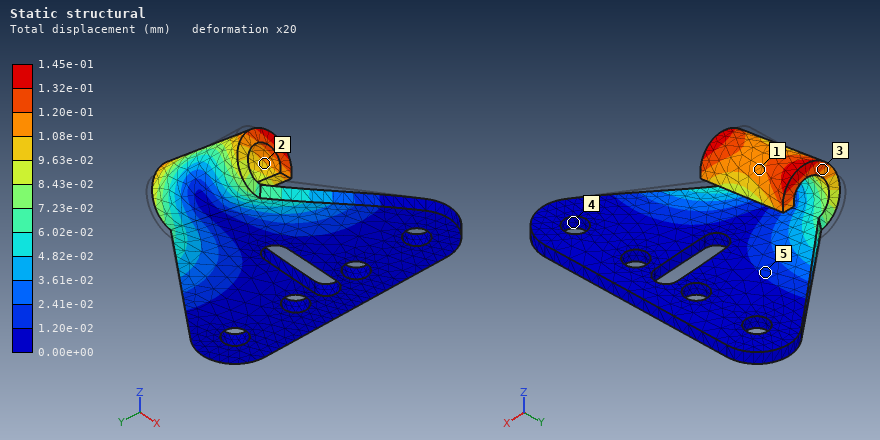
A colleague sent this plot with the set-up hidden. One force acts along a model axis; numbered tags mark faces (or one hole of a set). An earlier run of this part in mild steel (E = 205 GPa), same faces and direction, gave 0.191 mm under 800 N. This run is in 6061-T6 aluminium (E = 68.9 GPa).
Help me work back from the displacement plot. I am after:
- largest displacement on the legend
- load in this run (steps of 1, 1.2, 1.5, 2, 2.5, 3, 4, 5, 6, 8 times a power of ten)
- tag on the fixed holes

1.45e-01 mm
200 N
4
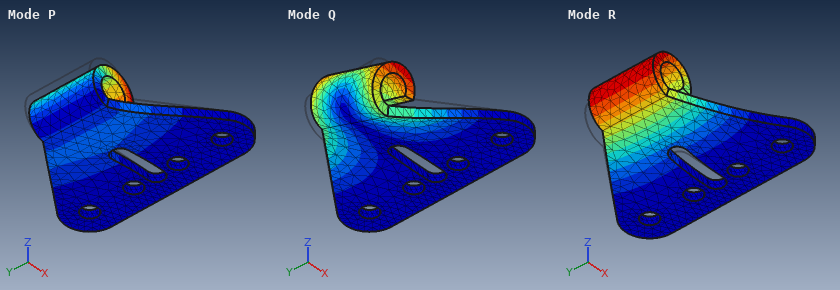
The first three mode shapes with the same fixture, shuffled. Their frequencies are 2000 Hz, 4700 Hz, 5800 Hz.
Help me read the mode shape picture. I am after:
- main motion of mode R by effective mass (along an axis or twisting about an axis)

along Z
